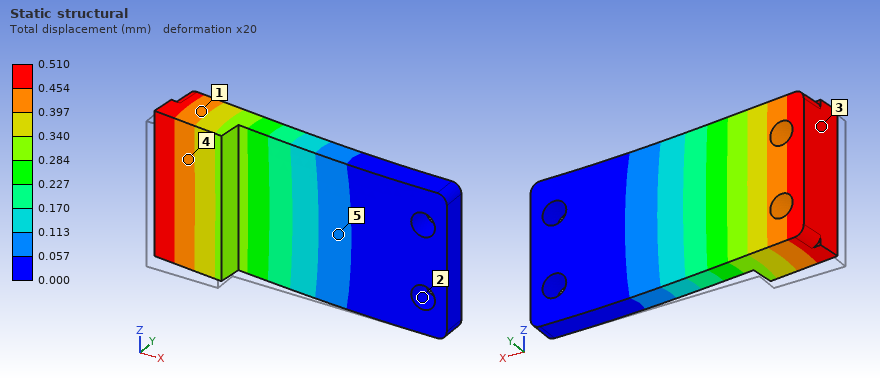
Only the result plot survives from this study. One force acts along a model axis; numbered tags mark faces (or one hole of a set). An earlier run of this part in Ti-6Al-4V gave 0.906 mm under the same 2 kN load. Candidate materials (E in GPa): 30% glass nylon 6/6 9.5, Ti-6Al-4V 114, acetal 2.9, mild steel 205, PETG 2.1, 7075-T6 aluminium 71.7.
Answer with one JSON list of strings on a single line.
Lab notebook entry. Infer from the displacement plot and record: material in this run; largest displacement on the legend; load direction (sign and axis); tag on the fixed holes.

["mild steel", "0.510 mm", "+Y", "2"]
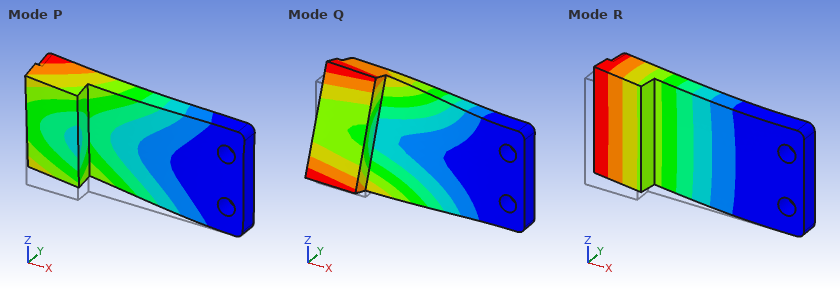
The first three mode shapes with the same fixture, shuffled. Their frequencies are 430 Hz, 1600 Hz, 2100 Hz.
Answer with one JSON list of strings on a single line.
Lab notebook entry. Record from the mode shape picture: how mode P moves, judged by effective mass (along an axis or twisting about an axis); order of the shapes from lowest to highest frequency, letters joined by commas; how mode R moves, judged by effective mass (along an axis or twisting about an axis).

["along Z", "R, Q, P", "along Y"]
